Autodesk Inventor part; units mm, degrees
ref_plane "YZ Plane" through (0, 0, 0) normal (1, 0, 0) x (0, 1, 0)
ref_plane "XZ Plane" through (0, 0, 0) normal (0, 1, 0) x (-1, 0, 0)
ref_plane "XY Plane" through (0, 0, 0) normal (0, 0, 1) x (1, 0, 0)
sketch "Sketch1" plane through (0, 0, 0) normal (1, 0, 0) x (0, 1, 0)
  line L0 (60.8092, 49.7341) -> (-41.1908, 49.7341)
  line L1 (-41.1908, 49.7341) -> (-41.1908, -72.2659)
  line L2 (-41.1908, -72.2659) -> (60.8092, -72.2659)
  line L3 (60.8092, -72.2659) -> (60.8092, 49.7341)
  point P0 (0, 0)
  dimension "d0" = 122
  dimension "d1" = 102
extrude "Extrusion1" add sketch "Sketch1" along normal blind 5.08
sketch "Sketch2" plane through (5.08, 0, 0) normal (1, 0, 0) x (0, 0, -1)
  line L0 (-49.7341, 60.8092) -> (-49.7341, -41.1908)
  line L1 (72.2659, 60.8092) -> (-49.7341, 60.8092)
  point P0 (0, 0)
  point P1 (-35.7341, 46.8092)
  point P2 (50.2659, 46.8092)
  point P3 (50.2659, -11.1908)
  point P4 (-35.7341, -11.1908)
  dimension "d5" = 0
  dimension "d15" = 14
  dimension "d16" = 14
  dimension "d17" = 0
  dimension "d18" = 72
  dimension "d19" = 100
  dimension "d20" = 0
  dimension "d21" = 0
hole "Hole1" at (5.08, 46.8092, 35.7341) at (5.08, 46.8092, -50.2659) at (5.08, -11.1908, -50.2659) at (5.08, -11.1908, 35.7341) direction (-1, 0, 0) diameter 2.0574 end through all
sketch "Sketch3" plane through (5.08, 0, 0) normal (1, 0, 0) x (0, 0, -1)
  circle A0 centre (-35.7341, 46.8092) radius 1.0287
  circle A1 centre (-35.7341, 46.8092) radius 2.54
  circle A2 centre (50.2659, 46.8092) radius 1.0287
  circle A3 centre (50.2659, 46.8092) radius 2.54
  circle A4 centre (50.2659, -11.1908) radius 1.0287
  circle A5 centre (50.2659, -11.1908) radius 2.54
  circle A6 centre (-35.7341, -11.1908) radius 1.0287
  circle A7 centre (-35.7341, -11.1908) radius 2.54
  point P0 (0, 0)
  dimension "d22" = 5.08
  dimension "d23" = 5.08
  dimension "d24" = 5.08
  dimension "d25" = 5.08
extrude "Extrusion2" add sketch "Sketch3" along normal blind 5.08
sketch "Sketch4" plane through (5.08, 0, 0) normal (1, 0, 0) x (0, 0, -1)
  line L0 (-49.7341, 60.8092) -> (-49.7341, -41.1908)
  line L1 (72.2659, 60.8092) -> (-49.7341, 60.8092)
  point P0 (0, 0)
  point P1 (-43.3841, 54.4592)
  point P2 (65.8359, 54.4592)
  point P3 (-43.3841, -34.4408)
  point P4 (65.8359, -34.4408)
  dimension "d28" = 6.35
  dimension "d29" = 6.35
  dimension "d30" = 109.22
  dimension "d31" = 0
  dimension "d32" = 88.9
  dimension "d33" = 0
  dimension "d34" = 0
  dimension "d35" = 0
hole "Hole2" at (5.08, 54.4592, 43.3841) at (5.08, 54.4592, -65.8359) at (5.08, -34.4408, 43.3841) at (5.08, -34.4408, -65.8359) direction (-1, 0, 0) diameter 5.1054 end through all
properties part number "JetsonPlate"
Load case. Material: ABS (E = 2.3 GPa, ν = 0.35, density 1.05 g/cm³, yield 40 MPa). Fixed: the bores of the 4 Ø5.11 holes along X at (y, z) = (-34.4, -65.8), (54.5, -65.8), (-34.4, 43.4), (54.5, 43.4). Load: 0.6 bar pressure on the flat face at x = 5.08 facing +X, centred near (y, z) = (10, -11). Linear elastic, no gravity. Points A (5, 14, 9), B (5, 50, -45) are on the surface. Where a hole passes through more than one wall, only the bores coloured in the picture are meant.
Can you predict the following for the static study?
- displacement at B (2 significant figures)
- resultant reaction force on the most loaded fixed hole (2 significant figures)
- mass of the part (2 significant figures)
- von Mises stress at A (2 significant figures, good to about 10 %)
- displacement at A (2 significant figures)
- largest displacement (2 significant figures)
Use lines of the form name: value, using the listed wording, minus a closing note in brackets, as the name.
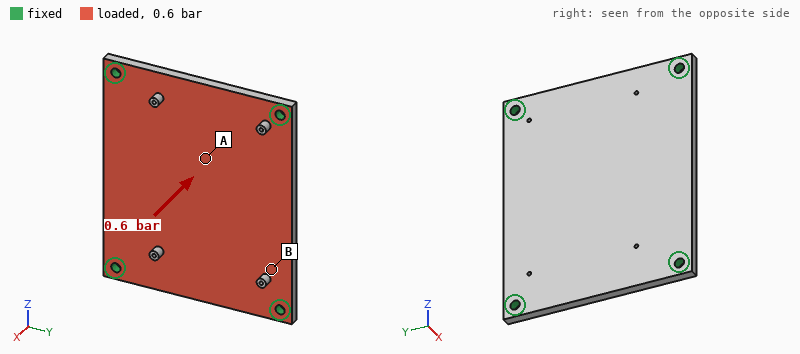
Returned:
displacement at B: 0.66 mm
resultant reaction force on the most loaded fixed hole: 190 N
mass of the part: 66 g
von Mises stress at A: 7.0 MPa
displacement at A: 1.6 mm
largest displacement: 1.8 mm
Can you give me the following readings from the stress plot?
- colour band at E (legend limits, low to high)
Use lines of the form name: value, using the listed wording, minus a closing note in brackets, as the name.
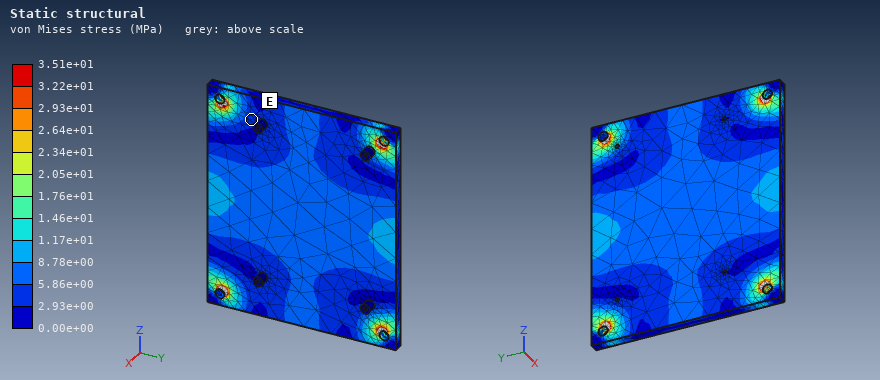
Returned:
colour band at E: 2.93e+00 to 5.86e+00 MPa
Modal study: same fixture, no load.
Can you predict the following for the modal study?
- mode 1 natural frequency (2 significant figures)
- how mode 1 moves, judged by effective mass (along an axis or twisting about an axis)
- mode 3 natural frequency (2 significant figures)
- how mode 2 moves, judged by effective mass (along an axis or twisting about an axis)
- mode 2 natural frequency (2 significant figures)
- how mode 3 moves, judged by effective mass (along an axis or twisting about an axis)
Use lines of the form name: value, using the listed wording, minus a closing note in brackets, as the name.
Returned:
mode 1 natural frequency: 470 Hz
how mode 1 moves, judged by effective mass: along X
mode 3 natural frequency: 970 Hz
how mode 2 moves, judged by effective mass: twisting about Z
mode 2 natural frequency: 770 Hz
how mode 3 moves, judged by effective mass: twisting about Y
